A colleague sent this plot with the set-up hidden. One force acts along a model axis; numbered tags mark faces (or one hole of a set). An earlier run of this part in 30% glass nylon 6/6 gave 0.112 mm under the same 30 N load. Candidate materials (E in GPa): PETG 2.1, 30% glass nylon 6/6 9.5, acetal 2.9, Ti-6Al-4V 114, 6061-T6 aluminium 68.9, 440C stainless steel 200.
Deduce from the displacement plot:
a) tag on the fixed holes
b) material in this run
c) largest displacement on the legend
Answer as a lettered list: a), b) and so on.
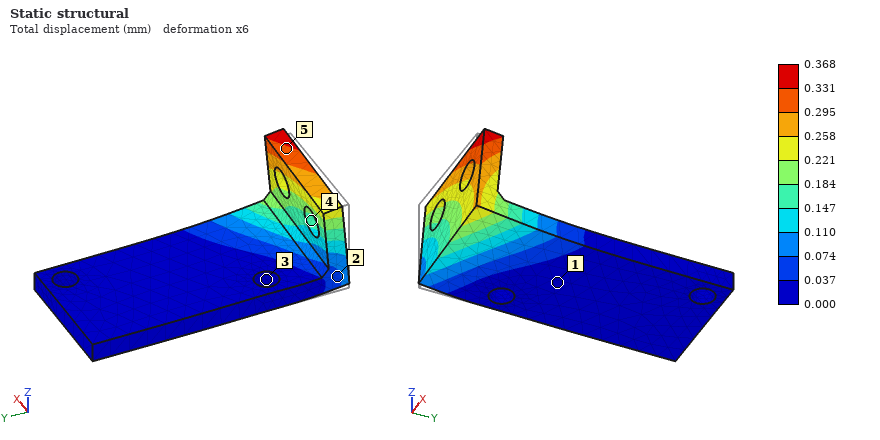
a) 3
b) acetal
c) 0.368 mm
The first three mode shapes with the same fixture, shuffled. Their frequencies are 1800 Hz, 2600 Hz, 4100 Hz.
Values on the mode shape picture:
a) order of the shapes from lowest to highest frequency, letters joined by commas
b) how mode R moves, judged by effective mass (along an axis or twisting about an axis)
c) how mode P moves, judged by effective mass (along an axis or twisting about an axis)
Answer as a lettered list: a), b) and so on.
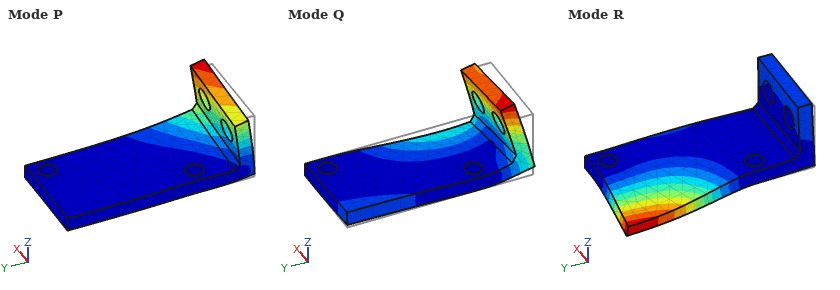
a) P, Q, R
b) along Z
c) along Z
